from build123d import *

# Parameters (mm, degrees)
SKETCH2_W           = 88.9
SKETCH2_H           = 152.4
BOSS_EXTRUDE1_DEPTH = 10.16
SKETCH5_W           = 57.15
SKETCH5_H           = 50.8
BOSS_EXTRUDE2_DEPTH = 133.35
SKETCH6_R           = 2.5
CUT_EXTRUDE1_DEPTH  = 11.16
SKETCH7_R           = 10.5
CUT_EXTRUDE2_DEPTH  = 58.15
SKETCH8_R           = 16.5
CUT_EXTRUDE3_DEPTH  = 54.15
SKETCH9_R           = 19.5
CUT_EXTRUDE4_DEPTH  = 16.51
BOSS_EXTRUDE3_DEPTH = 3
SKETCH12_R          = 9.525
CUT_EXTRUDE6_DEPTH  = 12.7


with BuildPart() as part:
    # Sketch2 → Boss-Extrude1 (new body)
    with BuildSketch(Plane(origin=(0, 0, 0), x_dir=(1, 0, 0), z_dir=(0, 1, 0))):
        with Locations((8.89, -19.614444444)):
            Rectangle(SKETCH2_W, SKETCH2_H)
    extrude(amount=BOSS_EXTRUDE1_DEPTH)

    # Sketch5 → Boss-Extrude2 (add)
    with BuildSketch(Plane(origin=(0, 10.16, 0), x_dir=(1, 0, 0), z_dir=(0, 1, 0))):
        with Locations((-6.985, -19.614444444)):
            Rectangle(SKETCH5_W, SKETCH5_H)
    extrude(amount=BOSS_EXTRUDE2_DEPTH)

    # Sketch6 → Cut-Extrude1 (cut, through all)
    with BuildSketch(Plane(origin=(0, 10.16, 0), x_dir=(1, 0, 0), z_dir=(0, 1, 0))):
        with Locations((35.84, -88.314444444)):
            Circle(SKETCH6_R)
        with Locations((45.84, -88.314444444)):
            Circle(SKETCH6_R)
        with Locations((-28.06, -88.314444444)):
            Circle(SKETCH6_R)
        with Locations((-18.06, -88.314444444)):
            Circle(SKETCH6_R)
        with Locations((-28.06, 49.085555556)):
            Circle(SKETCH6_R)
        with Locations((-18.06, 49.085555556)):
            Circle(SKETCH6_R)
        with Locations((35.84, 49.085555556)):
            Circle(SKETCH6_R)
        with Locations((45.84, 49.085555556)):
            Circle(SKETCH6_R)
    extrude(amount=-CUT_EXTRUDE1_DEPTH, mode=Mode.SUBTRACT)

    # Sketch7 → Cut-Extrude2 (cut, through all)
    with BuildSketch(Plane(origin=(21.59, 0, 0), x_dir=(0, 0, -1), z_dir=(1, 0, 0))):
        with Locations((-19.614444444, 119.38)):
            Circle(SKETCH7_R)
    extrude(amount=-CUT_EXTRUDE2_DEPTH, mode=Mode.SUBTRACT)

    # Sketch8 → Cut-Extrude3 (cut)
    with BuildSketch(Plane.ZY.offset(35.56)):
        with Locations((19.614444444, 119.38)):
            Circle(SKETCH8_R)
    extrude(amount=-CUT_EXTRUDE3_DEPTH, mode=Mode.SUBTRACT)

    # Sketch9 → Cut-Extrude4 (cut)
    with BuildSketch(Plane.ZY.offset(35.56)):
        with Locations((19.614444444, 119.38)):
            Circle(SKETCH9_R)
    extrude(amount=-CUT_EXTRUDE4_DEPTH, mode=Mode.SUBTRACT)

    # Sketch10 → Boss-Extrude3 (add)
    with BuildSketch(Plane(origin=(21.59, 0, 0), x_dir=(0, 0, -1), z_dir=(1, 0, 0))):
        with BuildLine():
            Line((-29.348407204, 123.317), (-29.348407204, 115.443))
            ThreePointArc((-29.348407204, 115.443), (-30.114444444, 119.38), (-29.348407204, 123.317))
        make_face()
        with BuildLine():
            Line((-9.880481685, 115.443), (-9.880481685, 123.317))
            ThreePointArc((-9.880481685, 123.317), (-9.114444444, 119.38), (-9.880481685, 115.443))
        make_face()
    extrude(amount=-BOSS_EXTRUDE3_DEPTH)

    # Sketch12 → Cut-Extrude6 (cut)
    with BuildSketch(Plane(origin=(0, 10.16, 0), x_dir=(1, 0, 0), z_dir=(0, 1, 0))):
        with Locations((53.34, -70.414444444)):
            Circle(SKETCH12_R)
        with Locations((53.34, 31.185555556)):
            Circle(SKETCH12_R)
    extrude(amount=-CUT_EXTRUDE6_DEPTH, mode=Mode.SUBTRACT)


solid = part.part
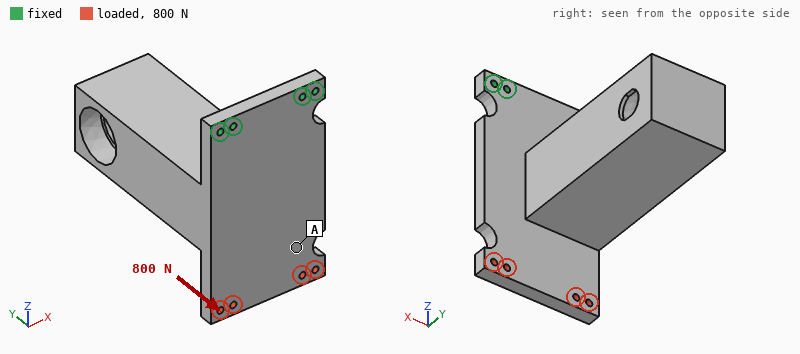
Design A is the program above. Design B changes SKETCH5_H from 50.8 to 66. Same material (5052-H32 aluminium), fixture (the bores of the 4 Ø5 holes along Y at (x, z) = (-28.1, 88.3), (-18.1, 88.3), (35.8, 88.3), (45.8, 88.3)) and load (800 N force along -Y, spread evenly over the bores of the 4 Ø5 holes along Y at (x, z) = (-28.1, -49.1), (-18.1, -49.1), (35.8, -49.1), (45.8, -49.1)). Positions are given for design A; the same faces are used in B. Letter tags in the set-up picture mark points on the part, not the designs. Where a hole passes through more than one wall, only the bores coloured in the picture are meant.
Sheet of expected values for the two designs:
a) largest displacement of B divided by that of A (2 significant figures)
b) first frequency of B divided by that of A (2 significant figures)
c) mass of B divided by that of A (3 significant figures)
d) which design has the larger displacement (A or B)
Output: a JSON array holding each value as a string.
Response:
["0.92", "0.91", "1.25", "A"]
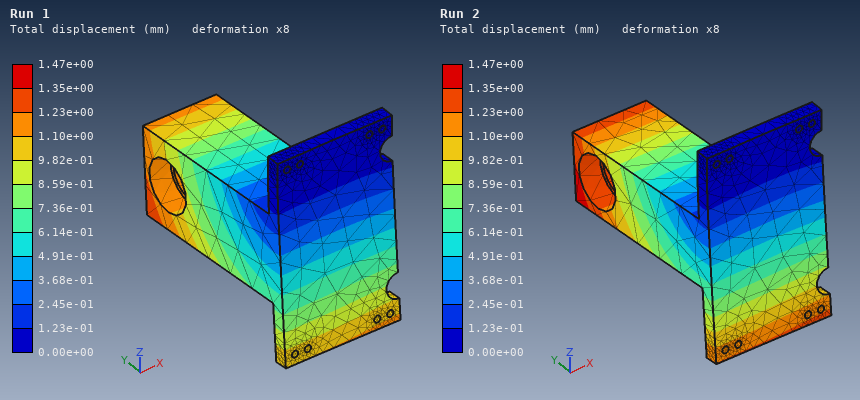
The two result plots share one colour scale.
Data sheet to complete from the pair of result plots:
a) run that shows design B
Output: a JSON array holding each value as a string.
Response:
["Run 1"]
